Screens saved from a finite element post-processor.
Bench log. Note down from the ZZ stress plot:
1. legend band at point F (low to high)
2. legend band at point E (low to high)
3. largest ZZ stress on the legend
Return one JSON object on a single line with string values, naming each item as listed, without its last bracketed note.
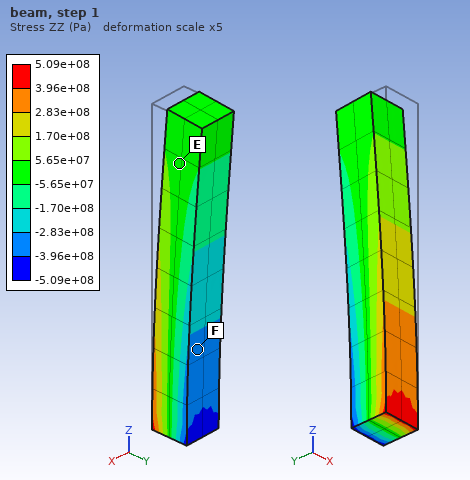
{"legend band at point F": "-3.96e+08 to -2.83e+08 Pa", "legend band at point E": "-5.65e+07 to 5.65e+07 Pa", "largest ZZ stress on the legend": "5.09e+08 Pa"}
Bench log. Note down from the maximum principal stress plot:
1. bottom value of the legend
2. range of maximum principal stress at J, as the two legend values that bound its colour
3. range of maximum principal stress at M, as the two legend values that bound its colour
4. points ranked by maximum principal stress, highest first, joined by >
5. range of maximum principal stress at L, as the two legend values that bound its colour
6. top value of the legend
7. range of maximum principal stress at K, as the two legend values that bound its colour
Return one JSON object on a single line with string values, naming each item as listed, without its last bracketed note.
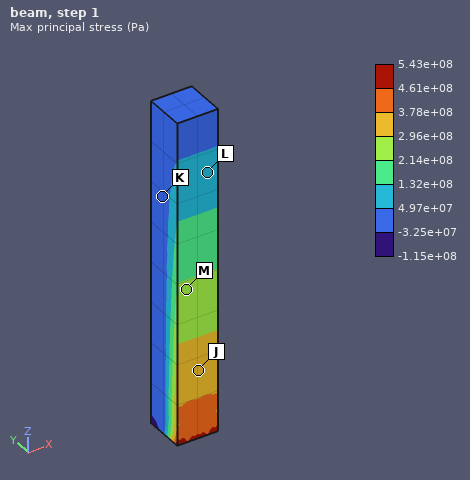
{"bottom value of the legend": "-1.15e+08 Pa", "range of maximum principal stress at J, as the two legend values that bound its colour": "2.96e+08 to 3.78e+08 Pa", "range of maximum principal stress at M, as the two legend values that bound its colour": "2.14e+08 to 2.96e+08 Pa", "points ranked by maximum principal stress, highest first, joined by >": "J > M > L > K", "range of maximum principal stress at L, as the two legend values that bound its colour": "4.97e+07 to 1.32e+08 Pa", "top value of the legend": "5.43e+08 Pa", "range of maximum principal stress at K, as the two legend values that bound its colour": "-3.25e+07 to 4.97e+07 Pa"}
